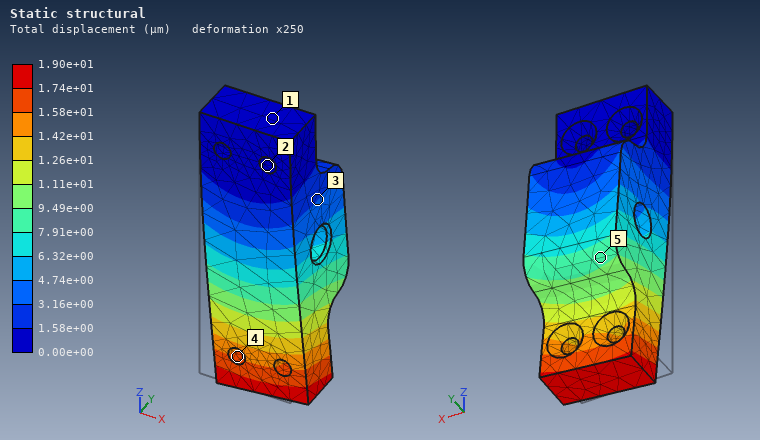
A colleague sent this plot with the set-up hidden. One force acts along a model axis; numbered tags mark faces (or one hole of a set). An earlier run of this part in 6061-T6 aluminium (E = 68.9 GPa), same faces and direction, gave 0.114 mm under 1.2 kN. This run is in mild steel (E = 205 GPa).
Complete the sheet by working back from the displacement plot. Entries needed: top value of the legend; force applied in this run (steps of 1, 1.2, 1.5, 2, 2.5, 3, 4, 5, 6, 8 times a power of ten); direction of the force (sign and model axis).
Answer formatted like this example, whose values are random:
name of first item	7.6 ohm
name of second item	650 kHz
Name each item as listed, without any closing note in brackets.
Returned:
top value of the legend	1.90e+01 µm
force applied in this run	600 N
direction of the force	+X
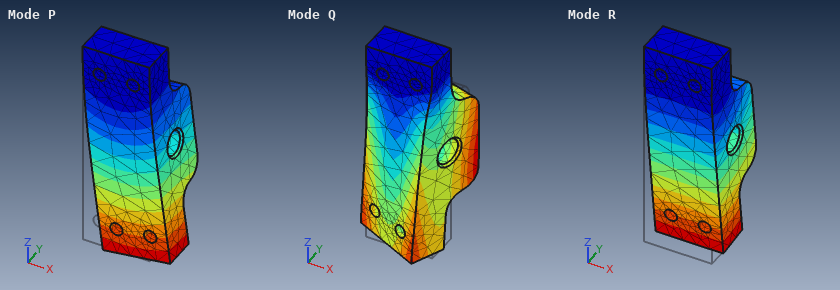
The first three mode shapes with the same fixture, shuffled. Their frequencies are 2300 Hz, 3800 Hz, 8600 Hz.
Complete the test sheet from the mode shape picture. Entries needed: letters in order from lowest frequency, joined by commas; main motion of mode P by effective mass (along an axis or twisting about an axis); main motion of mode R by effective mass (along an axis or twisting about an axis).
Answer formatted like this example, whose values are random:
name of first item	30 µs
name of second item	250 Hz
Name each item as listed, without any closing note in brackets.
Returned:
letters in order from lowest frequency, joined by commas	R, P, Q
main motion of mode P by effective mass	along X
main motion of mode R by effective mass	along Y
